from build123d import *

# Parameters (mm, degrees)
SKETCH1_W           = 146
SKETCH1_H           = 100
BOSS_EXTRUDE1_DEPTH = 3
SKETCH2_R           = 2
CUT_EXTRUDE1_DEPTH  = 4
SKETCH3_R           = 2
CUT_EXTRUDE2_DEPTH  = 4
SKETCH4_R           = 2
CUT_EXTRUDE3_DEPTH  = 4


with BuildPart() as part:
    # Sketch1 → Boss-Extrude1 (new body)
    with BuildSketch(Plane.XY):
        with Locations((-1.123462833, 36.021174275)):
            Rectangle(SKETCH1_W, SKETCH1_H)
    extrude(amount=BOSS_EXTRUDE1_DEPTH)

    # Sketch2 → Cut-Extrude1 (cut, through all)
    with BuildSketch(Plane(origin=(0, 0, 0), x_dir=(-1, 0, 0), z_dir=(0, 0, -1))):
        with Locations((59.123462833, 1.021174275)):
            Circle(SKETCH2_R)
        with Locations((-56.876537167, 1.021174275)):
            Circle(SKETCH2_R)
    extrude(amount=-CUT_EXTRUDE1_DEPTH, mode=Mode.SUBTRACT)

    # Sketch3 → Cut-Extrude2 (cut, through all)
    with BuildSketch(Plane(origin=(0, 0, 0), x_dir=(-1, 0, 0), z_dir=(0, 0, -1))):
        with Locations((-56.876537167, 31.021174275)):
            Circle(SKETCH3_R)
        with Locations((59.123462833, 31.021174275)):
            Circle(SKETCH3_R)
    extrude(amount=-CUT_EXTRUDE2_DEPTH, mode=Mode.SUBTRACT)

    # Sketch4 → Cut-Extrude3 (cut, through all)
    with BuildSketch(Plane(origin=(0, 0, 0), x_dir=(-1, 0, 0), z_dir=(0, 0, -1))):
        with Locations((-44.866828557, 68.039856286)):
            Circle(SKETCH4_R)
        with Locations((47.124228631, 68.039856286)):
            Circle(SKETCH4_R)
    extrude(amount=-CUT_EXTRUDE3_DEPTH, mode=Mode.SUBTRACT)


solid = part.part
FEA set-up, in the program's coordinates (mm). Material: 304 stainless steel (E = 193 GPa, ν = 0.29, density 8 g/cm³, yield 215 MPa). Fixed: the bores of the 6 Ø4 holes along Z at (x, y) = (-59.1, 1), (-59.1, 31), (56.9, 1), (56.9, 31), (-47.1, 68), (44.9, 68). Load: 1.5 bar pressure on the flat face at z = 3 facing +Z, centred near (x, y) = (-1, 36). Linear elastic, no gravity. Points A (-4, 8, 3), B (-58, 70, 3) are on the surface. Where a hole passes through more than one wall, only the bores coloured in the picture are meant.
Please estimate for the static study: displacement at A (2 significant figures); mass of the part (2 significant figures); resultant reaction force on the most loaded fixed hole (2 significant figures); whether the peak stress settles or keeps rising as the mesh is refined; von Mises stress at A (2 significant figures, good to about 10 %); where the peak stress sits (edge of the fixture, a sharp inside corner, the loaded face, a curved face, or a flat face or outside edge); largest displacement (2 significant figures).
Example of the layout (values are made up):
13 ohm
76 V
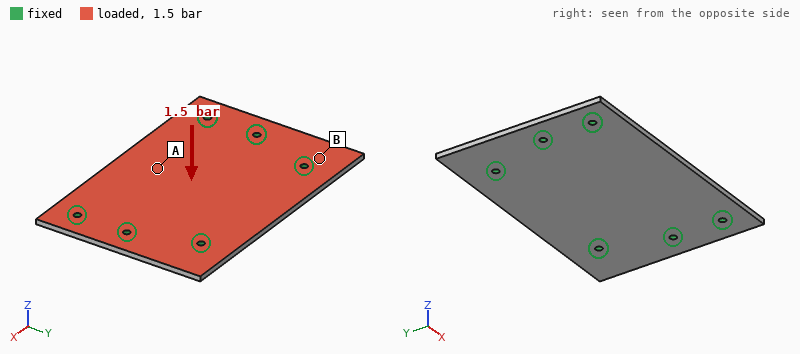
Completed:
0.15 mm
350 g
460 N
keeps rising
47 MPa
edge of the fixture
0.18 mm
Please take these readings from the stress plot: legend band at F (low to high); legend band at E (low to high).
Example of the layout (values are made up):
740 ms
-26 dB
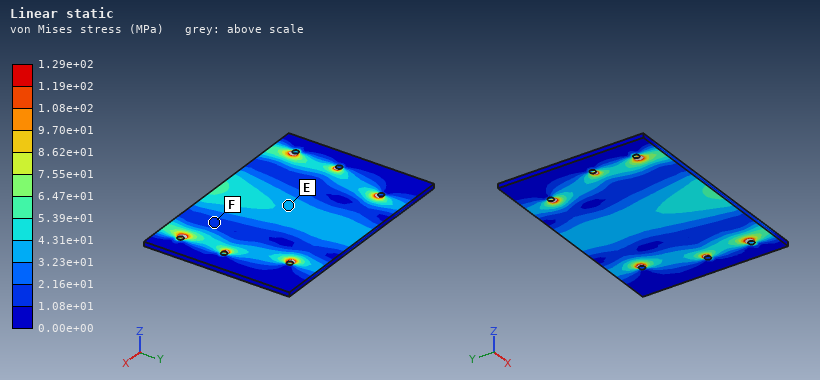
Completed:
1.08e+01 to 2.16e+01 MPa
3.23e+01 to 4.31e+01 MPa
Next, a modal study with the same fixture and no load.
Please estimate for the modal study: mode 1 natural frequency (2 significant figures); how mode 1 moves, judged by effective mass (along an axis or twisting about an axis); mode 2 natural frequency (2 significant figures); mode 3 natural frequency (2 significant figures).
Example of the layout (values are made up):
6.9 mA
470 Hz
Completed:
1200 Hz
along Z
1800 Hz
2700 Hz
